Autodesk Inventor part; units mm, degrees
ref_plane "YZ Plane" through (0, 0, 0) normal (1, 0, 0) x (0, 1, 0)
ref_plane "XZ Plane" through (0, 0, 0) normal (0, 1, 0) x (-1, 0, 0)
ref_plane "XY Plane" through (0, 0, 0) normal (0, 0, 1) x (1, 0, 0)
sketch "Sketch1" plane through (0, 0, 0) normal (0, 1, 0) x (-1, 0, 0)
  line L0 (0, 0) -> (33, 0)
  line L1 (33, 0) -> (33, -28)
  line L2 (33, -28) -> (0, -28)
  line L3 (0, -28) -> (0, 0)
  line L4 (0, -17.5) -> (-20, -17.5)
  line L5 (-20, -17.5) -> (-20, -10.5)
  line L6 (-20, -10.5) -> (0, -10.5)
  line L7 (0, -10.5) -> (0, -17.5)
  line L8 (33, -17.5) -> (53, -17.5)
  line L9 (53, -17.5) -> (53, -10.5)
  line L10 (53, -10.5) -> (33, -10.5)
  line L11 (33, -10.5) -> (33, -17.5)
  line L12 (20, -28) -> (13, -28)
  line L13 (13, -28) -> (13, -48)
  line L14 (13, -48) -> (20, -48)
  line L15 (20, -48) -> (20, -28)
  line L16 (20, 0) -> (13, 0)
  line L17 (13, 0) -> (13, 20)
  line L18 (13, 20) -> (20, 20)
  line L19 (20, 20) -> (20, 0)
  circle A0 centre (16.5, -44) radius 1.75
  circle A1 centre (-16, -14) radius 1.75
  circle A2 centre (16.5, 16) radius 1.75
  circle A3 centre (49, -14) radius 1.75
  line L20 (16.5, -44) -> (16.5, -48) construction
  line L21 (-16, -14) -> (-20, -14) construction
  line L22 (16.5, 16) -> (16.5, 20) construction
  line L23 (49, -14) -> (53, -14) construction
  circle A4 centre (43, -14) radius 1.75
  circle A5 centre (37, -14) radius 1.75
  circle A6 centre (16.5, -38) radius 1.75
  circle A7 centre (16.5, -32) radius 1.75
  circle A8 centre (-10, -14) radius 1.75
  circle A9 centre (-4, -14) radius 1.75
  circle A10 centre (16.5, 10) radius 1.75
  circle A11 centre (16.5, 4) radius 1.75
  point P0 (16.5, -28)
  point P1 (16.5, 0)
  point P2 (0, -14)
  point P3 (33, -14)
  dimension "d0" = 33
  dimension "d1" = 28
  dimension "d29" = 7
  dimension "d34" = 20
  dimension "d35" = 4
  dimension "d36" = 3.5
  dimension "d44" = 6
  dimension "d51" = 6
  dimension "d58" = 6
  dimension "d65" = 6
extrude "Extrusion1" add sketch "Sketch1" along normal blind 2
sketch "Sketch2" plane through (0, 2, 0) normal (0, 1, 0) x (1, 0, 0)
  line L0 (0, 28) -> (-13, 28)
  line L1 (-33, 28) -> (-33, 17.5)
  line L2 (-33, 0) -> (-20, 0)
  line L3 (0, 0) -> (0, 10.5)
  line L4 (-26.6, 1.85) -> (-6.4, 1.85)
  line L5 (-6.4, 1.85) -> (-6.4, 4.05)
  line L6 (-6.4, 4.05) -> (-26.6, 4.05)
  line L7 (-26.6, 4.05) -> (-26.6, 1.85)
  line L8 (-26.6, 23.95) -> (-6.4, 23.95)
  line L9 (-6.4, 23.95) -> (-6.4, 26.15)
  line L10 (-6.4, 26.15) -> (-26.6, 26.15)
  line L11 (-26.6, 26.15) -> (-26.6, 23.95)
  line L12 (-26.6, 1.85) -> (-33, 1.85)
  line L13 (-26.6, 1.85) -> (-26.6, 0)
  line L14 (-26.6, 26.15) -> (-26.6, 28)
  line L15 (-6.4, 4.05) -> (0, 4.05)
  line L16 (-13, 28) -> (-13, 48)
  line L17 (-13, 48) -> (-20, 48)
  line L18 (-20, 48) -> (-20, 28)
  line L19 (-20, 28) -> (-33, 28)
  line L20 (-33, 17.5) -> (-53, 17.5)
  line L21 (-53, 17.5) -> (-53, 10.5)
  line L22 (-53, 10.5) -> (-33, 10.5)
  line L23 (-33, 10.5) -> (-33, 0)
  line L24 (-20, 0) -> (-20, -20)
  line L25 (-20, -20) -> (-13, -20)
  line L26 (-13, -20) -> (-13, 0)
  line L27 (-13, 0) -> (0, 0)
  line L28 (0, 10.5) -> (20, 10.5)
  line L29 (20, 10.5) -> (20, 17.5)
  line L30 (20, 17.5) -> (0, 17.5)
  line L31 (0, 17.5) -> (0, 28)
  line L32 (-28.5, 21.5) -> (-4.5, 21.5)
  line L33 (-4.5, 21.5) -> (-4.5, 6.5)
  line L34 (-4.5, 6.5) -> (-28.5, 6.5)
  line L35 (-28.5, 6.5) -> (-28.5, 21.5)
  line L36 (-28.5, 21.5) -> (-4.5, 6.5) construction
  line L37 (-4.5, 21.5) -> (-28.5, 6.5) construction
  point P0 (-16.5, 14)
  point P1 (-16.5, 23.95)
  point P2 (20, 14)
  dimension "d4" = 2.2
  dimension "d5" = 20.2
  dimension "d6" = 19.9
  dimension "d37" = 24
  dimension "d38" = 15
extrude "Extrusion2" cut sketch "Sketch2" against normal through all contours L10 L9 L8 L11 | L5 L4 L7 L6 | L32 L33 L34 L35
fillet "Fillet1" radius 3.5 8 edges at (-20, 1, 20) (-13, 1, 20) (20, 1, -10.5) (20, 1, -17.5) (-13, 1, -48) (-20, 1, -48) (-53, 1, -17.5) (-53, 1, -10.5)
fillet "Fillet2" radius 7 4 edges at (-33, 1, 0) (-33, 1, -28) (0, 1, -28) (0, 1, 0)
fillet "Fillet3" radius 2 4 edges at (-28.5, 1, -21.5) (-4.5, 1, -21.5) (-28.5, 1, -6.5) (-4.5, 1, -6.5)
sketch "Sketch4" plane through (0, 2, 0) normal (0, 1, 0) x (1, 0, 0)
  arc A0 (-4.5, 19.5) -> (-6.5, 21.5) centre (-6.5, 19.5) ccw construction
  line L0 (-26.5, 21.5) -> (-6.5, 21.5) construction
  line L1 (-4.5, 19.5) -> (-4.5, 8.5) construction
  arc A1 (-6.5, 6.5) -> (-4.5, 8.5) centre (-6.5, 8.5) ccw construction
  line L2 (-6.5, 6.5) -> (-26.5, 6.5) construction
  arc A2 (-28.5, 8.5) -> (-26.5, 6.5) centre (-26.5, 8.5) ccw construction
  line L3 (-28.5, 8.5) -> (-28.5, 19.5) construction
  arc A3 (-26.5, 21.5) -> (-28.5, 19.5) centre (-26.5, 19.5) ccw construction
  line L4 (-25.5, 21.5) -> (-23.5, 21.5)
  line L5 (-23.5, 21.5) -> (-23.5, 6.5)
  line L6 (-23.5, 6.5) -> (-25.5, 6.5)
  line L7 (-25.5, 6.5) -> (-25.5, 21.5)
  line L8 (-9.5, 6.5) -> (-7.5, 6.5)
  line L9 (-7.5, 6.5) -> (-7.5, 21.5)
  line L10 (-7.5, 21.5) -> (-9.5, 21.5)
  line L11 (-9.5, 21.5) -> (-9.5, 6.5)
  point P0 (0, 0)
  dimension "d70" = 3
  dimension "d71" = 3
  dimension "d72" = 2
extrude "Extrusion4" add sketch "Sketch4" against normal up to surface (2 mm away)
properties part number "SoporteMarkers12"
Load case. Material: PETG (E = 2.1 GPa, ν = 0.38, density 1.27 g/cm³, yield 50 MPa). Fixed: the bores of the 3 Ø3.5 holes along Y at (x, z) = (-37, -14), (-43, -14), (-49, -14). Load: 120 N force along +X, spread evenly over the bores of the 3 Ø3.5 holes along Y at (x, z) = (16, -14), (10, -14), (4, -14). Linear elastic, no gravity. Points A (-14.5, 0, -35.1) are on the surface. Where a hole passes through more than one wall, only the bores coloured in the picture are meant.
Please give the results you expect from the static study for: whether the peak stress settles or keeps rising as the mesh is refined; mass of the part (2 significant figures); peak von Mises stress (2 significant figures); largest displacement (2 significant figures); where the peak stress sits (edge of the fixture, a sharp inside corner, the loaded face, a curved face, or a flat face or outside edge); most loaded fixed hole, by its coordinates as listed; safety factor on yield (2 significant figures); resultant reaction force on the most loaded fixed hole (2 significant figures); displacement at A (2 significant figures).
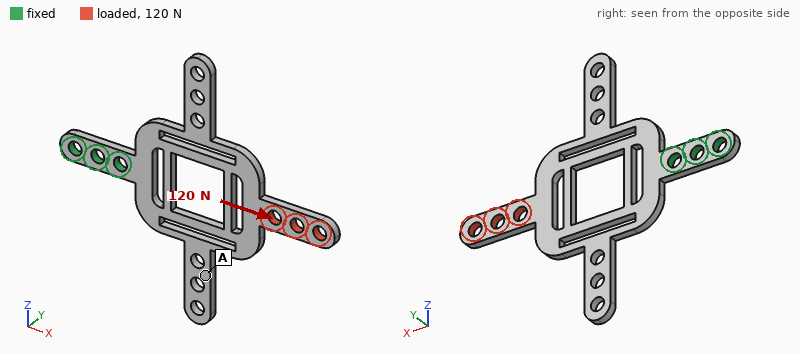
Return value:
settles
2.3 g
47 MPa
0.51 mm
a curved face
(-37, -14)
1.1
110 N
0.25 mm
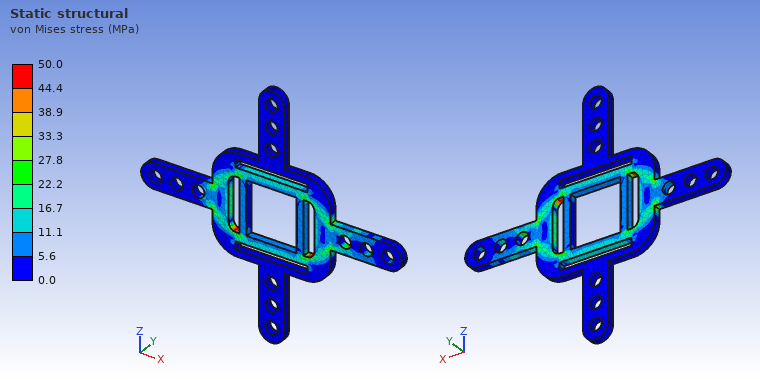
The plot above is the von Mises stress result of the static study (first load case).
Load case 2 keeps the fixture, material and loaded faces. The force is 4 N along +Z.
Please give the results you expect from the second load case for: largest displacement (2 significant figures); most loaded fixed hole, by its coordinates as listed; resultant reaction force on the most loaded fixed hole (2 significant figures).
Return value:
1.1 mm
(-37, -14)
9.8 N
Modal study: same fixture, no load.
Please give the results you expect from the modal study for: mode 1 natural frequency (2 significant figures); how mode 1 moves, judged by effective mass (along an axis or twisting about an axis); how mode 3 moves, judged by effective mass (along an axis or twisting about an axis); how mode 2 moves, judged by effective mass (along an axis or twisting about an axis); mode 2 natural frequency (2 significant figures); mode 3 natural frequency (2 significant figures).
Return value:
130 Hz
along Y
along Z
twisting about X
220 Hz
340 Hz
